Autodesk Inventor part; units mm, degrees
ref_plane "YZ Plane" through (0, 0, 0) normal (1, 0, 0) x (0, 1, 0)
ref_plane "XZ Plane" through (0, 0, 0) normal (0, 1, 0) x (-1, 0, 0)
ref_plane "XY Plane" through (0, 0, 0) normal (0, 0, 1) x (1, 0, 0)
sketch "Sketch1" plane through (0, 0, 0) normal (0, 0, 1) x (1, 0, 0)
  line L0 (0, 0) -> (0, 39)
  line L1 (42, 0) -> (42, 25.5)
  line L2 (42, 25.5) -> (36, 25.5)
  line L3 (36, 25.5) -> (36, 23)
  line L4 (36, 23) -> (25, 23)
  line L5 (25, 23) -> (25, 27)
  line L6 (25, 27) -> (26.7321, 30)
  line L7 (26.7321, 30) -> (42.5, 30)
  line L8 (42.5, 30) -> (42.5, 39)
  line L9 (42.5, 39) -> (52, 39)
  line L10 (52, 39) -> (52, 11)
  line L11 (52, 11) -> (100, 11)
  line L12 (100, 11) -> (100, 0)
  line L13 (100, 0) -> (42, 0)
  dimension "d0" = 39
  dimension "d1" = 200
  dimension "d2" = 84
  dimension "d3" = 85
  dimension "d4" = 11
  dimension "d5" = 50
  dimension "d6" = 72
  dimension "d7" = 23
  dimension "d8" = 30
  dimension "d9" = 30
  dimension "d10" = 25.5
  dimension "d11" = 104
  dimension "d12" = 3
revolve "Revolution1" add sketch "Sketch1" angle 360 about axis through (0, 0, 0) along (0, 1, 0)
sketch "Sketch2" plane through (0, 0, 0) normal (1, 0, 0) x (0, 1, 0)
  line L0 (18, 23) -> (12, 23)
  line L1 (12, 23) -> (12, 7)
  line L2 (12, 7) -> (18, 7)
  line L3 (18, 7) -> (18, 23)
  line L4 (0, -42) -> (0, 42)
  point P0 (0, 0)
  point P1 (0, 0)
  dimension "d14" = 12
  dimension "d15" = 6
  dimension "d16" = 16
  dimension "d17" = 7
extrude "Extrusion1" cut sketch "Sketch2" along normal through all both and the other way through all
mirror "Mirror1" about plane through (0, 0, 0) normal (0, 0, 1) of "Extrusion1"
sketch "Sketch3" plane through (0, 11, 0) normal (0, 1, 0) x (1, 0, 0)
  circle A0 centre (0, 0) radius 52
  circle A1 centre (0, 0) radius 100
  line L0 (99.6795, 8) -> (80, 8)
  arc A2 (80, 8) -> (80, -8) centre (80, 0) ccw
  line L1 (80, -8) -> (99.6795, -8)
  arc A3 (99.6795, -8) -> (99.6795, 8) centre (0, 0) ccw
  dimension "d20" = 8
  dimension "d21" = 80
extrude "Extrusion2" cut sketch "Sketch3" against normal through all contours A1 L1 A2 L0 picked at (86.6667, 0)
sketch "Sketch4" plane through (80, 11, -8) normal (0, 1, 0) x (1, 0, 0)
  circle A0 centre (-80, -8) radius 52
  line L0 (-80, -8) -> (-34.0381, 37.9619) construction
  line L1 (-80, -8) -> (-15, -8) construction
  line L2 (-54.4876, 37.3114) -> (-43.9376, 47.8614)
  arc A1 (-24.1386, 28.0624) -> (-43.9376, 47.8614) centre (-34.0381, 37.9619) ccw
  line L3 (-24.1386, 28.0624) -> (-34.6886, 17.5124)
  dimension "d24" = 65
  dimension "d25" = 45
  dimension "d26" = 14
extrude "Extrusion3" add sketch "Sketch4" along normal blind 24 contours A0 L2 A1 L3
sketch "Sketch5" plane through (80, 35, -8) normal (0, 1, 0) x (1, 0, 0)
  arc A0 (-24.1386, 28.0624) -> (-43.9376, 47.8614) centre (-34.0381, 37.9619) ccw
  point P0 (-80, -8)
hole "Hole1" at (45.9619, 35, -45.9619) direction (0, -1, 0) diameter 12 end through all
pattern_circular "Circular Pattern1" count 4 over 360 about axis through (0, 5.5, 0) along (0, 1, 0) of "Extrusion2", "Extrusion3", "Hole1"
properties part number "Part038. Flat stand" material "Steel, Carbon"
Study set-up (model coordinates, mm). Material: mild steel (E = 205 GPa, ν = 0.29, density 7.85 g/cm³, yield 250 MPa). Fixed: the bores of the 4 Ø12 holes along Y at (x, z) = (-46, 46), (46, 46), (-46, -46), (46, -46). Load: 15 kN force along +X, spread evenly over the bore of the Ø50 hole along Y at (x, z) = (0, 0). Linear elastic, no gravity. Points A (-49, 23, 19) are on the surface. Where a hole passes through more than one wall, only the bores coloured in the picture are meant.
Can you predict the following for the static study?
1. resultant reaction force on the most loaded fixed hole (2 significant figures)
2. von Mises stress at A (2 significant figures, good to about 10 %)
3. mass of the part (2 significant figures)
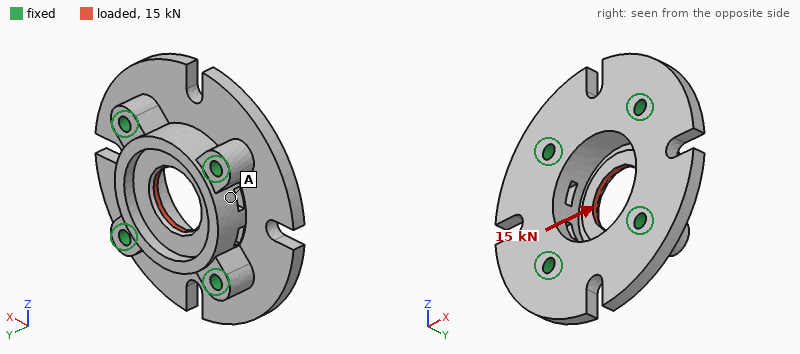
3.9 kN
6.0 MPa
3.3 kg
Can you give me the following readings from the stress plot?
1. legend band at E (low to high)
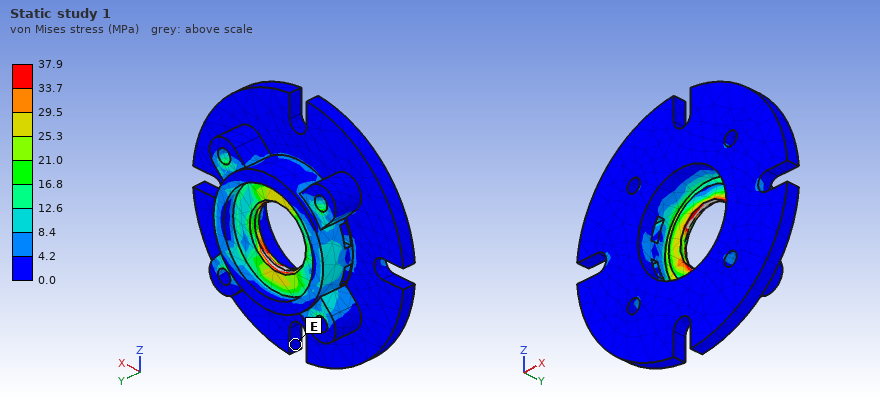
0.0 to 4.2 MPa
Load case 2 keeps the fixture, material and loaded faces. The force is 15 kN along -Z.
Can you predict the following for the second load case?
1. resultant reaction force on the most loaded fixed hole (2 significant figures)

3.9 kN
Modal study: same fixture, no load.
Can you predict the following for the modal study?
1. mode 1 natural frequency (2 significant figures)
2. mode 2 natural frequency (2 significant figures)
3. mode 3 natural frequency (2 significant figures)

4200 Hz
4400 Hz
4500 Hz
